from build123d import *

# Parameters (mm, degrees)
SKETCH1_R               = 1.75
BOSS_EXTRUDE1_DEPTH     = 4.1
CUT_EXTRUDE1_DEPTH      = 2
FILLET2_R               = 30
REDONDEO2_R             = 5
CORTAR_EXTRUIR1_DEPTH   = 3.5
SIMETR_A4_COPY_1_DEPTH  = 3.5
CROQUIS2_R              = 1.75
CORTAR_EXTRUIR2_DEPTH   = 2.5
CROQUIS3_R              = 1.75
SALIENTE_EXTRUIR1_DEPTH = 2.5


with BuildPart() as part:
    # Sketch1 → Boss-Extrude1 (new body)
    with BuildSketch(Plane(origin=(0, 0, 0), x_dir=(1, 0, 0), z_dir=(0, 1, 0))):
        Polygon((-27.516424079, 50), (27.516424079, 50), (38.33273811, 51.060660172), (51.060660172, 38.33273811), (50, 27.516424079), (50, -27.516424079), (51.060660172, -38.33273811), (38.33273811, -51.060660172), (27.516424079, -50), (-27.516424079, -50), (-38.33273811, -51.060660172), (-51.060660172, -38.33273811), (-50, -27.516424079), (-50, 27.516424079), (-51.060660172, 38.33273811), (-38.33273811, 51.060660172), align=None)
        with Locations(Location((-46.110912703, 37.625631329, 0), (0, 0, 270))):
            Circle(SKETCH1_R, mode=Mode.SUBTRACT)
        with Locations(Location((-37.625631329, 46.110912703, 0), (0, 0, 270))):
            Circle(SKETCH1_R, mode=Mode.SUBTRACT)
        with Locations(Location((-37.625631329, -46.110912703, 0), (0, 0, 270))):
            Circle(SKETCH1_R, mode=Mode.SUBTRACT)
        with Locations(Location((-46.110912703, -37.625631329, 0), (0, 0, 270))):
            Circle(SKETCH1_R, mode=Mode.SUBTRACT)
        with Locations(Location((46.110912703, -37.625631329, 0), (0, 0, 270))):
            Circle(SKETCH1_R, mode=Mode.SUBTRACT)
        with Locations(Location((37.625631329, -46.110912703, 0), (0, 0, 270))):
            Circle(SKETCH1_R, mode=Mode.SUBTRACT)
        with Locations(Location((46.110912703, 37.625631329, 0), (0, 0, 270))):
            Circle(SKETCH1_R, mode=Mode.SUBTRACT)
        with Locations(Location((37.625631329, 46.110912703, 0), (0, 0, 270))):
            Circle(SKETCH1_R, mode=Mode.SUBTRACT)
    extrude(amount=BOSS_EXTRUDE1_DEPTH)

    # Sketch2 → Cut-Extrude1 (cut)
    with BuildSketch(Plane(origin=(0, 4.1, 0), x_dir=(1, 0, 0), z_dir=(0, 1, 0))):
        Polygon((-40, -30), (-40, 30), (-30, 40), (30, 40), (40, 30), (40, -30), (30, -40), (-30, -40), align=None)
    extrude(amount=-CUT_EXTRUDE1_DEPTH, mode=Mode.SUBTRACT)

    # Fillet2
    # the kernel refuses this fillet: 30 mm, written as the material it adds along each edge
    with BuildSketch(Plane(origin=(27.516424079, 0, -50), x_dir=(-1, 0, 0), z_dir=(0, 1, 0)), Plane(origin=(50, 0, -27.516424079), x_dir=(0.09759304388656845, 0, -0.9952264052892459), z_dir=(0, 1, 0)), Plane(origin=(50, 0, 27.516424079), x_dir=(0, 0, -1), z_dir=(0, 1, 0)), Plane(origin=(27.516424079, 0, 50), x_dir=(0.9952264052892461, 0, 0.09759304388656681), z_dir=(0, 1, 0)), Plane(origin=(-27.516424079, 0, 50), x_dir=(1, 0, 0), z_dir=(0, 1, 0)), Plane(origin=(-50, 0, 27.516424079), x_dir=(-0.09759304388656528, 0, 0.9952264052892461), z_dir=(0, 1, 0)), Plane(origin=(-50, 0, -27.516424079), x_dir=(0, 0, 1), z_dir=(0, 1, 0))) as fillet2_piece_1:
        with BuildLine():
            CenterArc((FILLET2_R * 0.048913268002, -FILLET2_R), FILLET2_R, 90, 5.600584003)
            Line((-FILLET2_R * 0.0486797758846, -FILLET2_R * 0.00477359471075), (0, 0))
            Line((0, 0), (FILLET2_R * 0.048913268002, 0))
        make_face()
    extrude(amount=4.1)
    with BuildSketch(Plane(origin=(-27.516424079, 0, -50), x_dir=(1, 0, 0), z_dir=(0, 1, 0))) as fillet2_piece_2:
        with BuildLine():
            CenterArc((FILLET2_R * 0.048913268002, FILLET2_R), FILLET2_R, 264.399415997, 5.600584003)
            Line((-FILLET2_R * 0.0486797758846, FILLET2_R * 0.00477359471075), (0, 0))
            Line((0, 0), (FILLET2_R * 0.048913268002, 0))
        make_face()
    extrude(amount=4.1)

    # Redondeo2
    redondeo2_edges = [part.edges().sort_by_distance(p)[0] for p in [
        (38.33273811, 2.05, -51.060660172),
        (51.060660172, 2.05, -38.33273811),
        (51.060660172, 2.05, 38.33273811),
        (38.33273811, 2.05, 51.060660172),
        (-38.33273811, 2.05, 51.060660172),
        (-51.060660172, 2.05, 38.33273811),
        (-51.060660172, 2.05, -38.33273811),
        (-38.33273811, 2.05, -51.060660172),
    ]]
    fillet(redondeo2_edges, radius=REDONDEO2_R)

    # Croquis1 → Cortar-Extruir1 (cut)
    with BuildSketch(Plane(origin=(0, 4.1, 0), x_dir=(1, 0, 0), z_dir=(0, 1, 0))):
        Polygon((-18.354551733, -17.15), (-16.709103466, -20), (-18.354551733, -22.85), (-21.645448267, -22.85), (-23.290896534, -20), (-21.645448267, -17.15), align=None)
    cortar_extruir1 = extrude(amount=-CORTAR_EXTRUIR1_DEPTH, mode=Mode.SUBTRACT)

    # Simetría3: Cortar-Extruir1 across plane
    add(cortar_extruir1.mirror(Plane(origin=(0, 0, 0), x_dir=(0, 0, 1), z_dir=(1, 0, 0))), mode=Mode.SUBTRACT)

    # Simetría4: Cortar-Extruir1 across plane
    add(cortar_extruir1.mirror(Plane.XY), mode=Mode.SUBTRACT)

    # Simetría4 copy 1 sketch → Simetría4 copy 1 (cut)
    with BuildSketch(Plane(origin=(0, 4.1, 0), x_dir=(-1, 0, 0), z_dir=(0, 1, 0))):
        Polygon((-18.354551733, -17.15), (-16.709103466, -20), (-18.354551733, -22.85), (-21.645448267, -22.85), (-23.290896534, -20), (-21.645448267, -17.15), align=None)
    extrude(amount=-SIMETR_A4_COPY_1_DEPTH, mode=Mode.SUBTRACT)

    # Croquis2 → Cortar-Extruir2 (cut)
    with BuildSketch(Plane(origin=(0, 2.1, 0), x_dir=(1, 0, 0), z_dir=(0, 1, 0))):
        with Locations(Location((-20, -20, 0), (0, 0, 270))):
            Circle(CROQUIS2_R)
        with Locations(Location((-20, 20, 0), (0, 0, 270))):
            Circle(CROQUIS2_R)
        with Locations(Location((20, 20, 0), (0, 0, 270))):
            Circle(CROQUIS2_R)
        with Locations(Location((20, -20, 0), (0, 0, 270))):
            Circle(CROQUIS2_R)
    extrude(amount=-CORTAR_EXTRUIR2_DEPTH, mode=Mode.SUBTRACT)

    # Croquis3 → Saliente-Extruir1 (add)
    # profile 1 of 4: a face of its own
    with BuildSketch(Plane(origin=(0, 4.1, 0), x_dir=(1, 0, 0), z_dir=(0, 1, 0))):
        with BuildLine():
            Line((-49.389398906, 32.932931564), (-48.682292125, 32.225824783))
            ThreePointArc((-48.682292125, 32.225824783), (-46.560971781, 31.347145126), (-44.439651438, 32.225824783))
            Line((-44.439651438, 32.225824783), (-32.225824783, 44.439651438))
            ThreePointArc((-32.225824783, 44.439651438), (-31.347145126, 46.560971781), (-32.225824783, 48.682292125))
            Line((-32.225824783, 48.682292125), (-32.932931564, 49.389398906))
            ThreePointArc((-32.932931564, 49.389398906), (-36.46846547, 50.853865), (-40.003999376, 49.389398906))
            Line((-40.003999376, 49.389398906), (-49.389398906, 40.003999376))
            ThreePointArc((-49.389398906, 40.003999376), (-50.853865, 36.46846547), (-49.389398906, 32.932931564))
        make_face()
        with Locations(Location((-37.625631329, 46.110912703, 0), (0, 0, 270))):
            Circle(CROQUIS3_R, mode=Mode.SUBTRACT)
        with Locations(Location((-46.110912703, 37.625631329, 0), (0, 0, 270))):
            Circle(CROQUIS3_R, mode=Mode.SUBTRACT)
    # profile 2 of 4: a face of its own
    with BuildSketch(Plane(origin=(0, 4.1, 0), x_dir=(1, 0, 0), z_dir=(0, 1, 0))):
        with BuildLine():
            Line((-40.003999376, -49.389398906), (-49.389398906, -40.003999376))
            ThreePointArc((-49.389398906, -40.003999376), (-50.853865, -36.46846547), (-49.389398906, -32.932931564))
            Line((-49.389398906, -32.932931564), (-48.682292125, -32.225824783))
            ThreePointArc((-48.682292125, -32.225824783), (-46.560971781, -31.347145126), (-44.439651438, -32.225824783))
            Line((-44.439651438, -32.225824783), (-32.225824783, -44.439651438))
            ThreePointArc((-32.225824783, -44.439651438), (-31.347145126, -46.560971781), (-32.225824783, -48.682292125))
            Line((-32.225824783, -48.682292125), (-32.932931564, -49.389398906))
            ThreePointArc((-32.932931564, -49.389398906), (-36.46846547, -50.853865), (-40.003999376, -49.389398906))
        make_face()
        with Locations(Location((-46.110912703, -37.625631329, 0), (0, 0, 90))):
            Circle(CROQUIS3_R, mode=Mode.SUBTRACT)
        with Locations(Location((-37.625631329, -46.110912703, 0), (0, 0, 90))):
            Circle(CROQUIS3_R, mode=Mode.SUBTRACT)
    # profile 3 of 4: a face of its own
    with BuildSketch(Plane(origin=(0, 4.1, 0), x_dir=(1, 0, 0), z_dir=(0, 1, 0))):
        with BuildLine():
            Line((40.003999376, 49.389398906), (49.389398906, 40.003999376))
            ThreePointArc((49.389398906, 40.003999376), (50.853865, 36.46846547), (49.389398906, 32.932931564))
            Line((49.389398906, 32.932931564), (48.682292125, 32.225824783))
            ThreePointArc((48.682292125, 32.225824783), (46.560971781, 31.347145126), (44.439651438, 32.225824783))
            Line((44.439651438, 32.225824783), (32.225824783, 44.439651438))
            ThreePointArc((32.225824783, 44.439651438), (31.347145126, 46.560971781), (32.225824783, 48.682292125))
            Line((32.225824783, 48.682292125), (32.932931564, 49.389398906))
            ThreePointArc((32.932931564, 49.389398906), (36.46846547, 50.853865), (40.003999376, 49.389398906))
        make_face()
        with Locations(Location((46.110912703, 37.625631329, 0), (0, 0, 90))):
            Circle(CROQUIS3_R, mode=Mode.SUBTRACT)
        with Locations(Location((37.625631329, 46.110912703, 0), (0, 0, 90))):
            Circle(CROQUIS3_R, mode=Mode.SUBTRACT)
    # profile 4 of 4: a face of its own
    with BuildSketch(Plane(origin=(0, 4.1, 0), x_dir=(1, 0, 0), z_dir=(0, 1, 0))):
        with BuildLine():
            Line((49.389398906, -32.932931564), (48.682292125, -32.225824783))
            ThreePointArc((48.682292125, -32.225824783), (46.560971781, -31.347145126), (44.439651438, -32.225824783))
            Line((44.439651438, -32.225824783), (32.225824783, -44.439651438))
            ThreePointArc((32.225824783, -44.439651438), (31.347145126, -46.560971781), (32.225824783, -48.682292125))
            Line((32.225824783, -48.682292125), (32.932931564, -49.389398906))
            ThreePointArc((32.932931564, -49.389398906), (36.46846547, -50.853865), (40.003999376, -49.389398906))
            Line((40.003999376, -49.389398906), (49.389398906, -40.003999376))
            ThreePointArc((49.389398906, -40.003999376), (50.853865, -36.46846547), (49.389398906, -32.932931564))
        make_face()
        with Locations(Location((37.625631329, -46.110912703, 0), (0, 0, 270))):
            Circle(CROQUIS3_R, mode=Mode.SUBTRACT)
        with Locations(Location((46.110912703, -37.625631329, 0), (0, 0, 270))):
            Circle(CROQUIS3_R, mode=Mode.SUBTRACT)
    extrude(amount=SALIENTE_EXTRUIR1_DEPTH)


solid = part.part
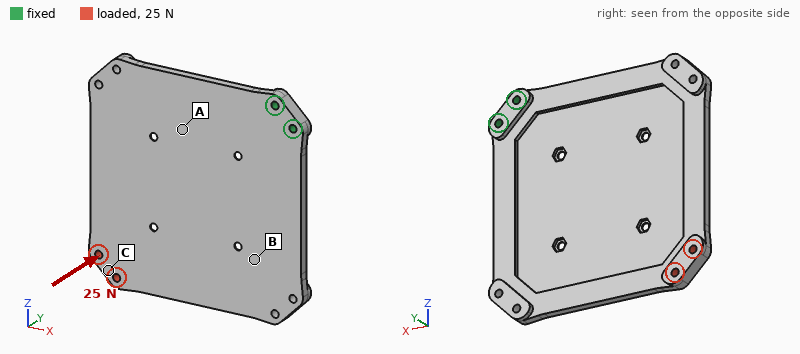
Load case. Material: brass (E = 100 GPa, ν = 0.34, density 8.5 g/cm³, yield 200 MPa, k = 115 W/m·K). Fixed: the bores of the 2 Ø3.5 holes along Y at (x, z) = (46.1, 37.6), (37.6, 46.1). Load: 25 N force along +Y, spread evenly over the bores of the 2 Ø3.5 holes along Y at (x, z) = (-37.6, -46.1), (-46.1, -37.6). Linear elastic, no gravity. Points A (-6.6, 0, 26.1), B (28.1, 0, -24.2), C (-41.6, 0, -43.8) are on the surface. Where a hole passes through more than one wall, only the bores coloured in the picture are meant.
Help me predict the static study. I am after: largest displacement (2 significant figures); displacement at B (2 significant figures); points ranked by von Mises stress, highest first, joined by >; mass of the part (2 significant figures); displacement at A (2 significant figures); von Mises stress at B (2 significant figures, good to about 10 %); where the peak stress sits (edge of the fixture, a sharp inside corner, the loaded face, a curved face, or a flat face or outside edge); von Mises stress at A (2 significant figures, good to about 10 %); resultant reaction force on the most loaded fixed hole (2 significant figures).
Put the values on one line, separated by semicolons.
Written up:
0.87 mm; 0.24 mm; A > B > C; 250 g; 0.16 mm; 6.4 MPa; a curved face; 11 MPa; 110 N
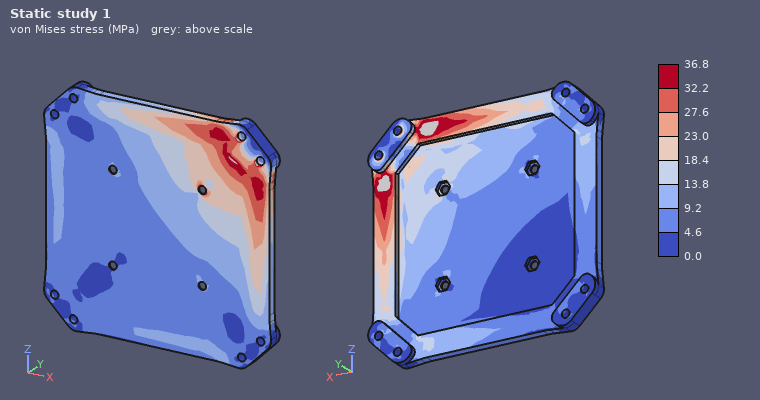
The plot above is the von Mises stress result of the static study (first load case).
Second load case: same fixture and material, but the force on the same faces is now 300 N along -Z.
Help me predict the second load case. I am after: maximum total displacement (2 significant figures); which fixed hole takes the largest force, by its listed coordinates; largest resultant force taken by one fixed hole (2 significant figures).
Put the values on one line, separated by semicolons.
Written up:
0.25 mm; (37.6, 46.1); 1.7 kN
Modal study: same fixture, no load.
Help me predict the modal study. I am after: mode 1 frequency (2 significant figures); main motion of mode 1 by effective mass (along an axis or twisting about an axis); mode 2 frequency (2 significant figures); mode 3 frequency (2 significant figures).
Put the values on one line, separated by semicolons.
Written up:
120 Hz; along Y; 240 Hz; 520 Hz
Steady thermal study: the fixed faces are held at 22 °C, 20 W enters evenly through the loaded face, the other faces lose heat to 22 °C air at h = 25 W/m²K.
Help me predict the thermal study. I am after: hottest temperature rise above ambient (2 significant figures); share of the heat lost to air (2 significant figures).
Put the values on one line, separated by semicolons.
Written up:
75 K; 70 %
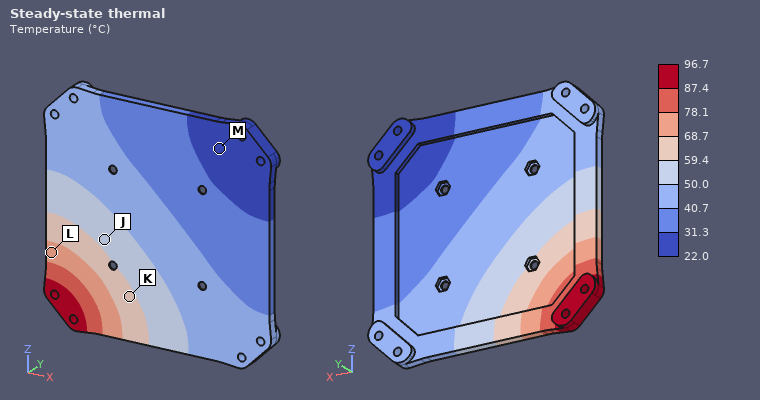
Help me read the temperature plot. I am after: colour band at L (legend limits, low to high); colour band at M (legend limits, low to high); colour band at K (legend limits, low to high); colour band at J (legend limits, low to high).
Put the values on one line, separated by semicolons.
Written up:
68.7 to 78.1 °C; 22.0 to 31.3 °C; 59.4 to 68.7 °C; 50.0 to 59.4 °C
